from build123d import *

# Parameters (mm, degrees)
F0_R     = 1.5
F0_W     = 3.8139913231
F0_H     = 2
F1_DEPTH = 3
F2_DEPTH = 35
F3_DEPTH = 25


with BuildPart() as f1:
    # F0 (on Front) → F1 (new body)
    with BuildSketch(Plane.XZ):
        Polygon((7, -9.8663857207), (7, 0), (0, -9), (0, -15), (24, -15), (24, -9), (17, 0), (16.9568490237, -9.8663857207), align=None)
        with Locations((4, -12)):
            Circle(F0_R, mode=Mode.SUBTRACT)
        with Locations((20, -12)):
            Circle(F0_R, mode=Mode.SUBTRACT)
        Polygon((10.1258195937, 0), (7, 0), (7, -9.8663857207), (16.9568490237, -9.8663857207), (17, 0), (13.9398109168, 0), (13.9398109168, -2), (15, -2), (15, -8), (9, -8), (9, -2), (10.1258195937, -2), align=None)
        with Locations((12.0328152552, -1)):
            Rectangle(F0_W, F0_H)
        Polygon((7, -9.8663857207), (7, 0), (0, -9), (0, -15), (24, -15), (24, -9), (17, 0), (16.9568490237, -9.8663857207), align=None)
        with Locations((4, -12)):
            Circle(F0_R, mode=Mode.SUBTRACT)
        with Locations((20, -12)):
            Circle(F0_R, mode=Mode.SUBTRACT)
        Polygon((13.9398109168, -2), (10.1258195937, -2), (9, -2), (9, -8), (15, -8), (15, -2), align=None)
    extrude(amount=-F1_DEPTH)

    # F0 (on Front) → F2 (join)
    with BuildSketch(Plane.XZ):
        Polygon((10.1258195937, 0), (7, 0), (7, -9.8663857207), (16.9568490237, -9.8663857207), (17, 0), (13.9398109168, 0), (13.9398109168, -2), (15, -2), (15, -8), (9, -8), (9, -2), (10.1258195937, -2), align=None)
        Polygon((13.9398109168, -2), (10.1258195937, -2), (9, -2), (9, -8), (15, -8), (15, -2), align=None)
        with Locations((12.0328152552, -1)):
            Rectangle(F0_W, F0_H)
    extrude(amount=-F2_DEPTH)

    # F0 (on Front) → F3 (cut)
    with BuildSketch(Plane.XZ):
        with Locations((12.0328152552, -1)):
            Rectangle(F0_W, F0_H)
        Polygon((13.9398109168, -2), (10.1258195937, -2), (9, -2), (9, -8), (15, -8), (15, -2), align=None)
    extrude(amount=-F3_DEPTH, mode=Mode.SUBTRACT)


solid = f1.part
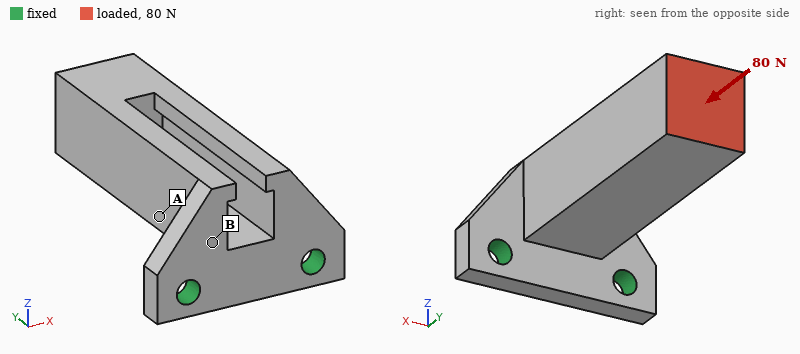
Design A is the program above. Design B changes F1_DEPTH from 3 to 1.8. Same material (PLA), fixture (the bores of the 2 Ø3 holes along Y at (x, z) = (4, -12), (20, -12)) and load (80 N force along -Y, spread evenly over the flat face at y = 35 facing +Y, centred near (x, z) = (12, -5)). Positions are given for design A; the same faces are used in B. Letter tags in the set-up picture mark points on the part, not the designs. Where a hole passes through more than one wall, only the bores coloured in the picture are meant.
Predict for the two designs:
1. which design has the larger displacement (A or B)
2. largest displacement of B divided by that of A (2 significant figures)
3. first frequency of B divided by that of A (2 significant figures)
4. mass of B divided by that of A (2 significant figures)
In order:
B
3.2
0.57
0.92
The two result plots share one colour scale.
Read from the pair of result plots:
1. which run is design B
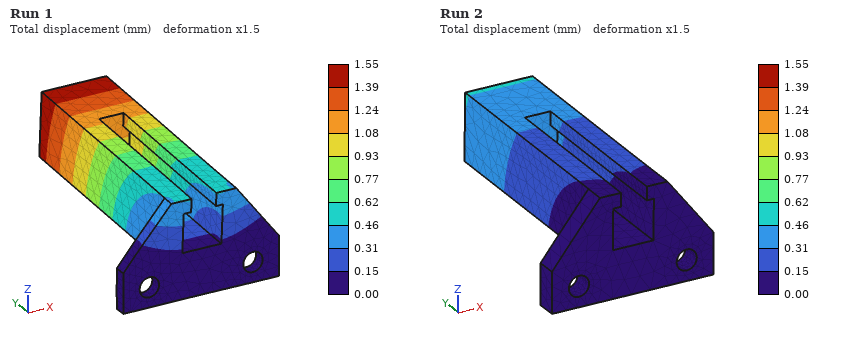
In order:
Run 1
